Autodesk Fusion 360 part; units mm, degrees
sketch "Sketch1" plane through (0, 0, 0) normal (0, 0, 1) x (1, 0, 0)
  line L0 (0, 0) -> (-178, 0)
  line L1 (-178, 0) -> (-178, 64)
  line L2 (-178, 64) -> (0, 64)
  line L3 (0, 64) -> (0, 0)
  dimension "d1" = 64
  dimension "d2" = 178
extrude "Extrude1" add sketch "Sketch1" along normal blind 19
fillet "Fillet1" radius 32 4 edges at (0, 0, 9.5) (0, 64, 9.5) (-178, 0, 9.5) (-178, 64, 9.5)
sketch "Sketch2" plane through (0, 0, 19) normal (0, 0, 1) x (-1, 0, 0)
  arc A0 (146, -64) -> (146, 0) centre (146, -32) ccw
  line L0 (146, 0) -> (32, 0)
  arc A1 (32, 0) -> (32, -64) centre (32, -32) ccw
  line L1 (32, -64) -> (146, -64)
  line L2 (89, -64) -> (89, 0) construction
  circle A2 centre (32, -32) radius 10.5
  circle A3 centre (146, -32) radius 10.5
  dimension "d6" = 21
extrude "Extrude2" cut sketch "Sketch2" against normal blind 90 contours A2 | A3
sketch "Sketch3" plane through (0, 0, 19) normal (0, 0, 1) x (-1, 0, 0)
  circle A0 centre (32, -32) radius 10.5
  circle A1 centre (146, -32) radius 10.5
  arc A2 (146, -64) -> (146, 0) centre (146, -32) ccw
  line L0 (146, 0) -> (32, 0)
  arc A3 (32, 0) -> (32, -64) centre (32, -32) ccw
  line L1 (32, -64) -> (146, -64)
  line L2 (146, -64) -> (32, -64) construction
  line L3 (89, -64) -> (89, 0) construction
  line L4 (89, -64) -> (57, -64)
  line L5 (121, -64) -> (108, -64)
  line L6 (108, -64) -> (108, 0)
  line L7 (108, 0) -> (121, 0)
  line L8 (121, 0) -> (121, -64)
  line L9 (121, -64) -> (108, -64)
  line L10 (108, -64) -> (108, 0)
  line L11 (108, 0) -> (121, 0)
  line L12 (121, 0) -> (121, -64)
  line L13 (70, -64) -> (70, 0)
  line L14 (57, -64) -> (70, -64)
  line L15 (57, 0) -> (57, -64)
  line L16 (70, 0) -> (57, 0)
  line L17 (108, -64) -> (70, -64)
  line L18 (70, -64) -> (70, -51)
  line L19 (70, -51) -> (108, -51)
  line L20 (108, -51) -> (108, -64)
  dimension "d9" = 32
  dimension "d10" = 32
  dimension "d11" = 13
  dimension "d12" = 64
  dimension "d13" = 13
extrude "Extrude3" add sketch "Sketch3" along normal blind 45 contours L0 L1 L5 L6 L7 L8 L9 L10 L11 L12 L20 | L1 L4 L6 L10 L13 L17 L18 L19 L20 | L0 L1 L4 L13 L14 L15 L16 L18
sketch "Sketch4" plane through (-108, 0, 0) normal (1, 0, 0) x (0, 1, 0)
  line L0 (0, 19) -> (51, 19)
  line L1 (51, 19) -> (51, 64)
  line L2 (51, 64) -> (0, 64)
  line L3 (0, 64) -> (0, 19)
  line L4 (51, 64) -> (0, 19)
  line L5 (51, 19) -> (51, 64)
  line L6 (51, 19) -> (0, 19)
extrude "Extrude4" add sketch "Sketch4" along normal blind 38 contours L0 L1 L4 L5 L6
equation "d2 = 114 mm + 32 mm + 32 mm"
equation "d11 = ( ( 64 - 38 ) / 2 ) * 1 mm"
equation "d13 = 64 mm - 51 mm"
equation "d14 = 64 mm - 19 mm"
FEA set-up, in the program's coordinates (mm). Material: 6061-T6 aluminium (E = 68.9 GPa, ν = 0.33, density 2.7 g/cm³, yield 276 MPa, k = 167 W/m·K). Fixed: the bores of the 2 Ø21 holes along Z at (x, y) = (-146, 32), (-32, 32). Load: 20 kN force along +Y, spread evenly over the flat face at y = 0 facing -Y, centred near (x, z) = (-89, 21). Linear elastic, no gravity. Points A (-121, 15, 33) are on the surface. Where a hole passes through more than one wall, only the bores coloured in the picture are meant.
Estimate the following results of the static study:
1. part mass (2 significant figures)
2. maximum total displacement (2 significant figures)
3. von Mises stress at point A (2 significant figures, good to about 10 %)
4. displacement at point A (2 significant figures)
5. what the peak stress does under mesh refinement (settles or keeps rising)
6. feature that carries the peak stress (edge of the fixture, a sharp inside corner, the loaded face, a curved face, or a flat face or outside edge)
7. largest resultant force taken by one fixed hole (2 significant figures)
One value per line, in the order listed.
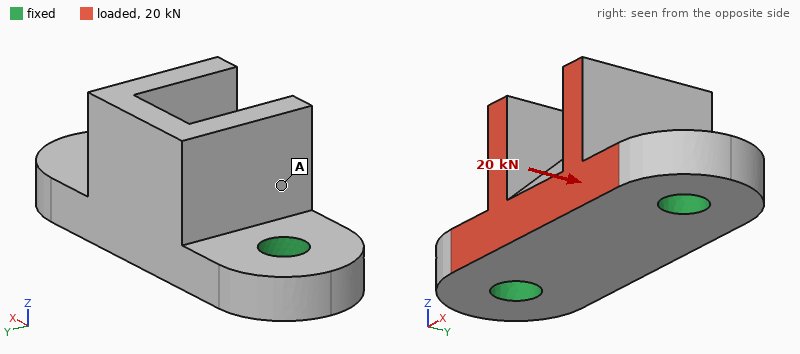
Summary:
880 g
61 µm
10 MPa
32 µm
keeps rising
edge of the fixture
10 kN
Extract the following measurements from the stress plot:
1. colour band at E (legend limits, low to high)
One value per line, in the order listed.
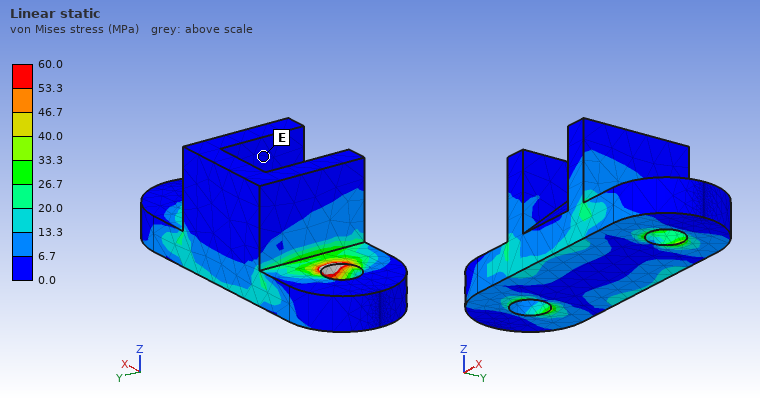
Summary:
0.0 to 6.7 MPa
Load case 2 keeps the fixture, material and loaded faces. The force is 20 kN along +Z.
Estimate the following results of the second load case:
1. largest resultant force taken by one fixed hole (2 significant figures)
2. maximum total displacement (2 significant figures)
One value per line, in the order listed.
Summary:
10 kN
0.13 mm
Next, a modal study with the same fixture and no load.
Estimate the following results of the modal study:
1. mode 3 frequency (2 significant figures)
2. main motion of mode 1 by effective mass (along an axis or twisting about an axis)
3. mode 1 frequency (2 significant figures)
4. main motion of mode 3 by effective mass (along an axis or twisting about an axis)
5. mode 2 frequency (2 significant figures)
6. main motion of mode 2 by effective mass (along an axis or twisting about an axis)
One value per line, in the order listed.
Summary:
7000 Hz
along Y
3400 Hz
along X
6100 Hz
along Z
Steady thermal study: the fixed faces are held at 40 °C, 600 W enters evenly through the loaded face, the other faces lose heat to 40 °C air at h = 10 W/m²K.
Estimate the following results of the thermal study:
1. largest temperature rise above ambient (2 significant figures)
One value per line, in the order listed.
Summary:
72 K
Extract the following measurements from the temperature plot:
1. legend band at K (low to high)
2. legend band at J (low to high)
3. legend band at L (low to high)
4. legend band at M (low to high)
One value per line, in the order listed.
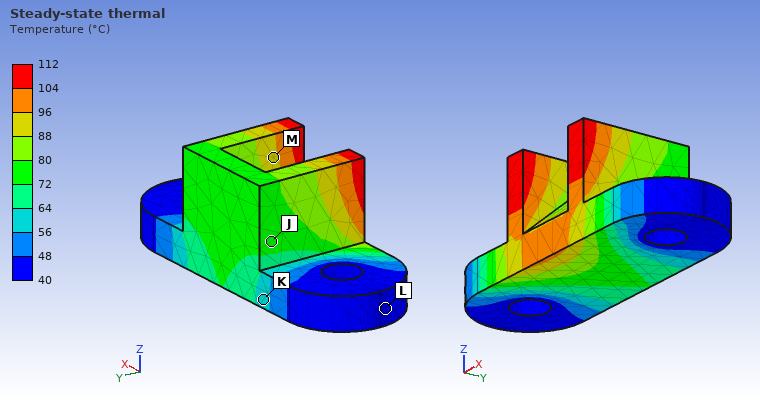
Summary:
56 to 64 °C
72 to 80 °C
40 to 48 °C
88 to 96 °C
